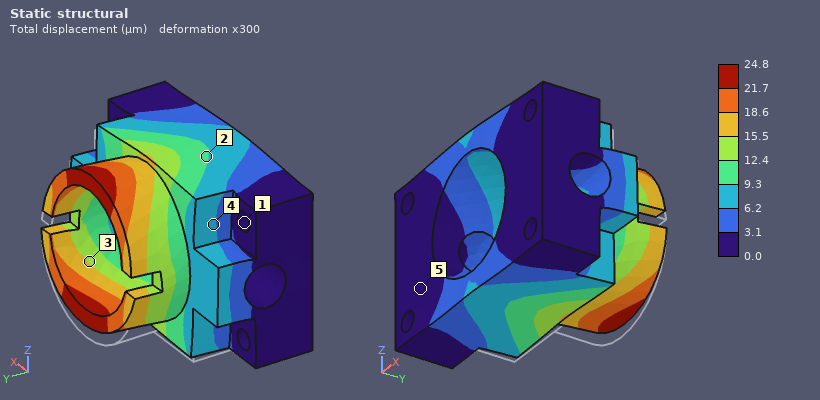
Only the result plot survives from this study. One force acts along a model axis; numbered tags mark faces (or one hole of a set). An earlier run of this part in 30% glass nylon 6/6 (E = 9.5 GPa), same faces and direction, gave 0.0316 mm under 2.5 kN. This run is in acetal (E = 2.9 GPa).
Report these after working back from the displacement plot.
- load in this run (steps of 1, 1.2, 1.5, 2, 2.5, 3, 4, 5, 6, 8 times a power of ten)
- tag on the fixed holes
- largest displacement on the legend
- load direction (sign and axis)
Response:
600 N
1
24.8 µm
+Z
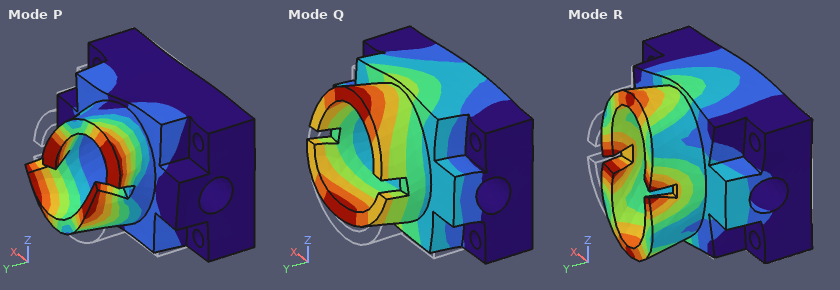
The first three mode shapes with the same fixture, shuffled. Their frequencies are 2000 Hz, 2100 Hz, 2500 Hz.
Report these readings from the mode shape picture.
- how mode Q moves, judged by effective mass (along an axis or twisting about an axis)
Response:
along Z
